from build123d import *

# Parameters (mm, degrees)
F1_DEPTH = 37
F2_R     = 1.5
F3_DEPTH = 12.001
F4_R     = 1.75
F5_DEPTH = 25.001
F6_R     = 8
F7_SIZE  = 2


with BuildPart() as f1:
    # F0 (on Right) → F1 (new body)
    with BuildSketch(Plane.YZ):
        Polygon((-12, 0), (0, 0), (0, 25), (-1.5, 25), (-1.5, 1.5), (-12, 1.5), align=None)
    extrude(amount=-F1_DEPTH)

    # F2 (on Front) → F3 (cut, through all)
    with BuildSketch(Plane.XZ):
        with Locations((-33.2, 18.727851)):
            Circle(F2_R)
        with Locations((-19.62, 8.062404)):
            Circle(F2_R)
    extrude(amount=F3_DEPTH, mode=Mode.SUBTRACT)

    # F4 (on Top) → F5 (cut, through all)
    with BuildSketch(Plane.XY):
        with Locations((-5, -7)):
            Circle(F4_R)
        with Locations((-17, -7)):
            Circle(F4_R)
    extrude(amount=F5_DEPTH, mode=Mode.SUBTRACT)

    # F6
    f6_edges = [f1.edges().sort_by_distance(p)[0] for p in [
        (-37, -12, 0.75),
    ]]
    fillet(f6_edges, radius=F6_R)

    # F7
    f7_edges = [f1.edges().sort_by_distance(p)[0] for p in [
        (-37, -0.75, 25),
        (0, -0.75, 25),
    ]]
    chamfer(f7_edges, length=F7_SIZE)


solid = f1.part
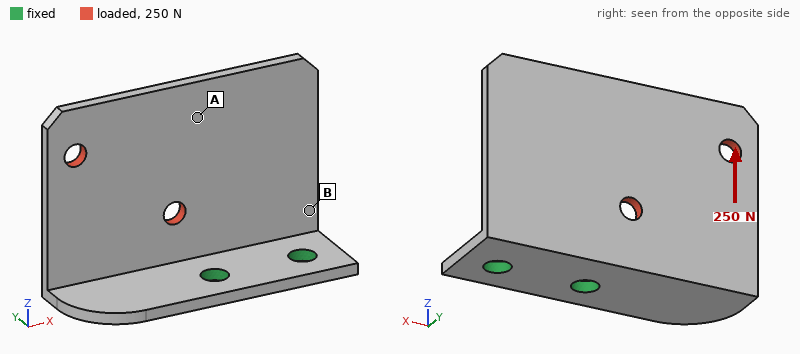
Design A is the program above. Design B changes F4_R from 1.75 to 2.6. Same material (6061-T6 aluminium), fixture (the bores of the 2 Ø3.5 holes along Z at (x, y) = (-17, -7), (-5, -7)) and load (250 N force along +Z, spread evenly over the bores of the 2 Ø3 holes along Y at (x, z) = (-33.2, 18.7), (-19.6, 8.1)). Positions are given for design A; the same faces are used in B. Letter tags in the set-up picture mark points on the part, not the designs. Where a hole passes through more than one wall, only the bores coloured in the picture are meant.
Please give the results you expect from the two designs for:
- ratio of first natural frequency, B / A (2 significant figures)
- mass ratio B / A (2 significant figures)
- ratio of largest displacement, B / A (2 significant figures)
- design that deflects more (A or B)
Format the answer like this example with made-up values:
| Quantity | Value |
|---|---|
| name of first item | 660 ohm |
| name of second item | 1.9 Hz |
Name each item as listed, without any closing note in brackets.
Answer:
| Quantity | Value |
|---|---|
| ratio of first natural frequency, B / A | 1.1 |
| mass ratio B / A | 0.98 |
| ratio of largest displacement, B / A | 0.67 |
| design that deflects more | A |
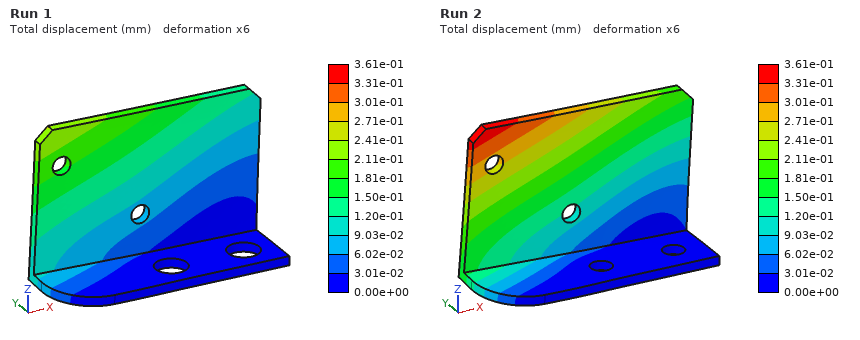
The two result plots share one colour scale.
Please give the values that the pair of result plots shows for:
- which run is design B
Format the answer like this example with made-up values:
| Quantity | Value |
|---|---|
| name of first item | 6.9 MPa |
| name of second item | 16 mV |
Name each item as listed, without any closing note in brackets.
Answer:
| Quantity | Value |
|---|---|
| which run is design B | Run 1 |
